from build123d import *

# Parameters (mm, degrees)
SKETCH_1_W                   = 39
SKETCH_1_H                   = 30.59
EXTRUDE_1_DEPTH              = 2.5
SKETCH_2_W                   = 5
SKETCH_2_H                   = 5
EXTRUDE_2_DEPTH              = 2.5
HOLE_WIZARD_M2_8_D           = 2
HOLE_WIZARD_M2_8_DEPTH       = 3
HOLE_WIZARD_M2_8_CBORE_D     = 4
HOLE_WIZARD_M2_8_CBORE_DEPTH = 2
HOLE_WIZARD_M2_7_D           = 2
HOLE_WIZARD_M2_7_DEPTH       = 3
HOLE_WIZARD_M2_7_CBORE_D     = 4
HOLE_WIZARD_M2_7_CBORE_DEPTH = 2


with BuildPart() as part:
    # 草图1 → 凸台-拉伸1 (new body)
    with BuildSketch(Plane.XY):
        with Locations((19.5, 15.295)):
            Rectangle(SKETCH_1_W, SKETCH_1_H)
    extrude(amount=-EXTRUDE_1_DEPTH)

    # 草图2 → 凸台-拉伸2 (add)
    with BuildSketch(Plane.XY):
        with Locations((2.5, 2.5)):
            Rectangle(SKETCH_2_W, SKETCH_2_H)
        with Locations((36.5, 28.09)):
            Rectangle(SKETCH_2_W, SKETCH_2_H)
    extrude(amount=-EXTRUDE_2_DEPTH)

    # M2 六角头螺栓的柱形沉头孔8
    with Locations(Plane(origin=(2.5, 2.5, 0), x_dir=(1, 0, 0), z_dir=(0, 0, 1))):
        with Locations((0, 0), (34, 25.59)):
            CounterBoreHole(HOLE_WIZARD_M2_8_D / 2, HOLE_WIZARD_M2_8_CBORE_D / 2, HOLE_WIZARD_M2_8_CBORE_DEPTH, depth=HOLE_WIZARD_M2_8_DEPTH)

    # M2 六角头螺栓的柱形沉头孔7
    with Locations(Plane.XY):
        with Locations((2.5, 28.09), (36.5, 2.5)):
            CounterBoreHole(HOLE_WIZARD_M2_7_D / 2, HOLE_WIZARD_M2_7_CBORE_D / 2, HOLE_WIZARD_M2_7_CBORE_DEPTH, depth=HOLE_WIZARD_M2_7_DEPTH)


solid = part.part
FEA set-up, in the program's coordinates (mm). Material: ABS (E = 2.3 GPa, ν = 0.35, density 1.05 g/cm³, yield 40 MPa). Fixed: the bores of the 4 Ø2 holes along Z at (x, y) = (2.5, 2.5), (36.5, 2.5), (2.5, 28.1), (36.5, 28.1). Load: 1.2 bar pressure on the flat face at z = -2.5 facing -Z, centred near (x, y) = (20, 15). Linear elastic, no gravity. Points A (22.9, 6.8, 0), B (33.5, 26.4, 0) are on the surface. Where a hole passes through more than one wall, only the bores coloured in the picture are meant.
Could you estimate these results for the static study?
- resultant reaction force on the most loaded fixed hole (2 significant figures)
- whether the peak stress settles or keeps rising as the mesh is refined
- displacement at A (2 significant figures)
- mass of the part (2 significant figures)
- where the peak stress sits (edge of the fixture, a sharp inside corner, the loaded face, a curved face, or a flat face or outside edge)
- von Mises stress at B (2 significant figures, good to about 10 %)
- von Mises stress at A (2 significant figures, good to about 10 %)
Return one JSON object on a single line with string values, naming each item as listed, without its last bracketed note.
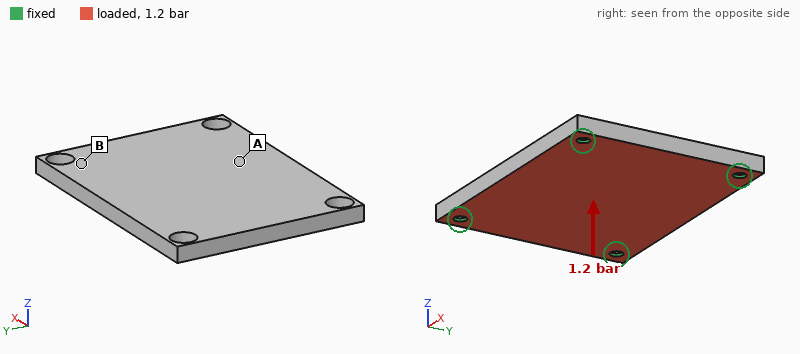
{"resultant reaction force on the most loaded fixed hole": "74 N", "whether the peak stress settles or keeps rising as the mesh is refined": "keeps rising", "displacement at A": "0.40 mm", "mass of the part": "3.0 g", "where the peak stress sits": "edge of the fixture", "von Mises stress at B": "5.1 MPa", "von Mises stress at A": "10 MPa"}
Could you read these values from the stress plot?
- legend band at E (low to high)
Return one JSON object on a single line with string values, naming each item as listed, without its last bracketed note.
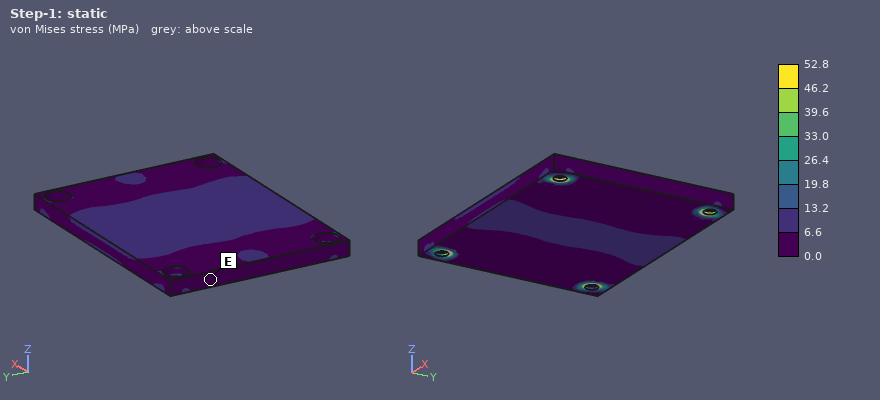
{"legend band at E": "0.0 to 6.6 MPa"}
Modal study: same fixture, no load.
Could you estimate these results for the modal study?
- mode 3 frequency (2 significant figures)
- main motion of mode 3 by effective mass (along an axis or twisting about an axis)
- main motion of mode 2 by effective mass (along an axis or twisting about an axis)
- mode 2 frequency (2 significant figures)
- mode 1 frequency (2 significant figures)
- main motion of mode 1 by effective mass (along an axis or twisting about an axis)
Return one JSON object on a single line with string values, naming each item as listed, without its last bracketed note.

{"mode 3 frequency": "3900 Hz", "main motion of mode 3 by effective mass": "twisting about Y", "main motion of mode 2 by effective mass": "twisting about X", "mode 2 frequency": "3000 Hz", "mode 1 frequency": "1900 Hz", "main motion of mode 1 by effective mass": "along Z"}
